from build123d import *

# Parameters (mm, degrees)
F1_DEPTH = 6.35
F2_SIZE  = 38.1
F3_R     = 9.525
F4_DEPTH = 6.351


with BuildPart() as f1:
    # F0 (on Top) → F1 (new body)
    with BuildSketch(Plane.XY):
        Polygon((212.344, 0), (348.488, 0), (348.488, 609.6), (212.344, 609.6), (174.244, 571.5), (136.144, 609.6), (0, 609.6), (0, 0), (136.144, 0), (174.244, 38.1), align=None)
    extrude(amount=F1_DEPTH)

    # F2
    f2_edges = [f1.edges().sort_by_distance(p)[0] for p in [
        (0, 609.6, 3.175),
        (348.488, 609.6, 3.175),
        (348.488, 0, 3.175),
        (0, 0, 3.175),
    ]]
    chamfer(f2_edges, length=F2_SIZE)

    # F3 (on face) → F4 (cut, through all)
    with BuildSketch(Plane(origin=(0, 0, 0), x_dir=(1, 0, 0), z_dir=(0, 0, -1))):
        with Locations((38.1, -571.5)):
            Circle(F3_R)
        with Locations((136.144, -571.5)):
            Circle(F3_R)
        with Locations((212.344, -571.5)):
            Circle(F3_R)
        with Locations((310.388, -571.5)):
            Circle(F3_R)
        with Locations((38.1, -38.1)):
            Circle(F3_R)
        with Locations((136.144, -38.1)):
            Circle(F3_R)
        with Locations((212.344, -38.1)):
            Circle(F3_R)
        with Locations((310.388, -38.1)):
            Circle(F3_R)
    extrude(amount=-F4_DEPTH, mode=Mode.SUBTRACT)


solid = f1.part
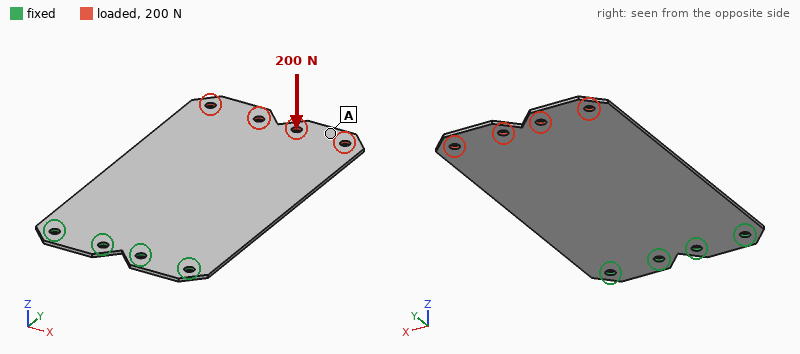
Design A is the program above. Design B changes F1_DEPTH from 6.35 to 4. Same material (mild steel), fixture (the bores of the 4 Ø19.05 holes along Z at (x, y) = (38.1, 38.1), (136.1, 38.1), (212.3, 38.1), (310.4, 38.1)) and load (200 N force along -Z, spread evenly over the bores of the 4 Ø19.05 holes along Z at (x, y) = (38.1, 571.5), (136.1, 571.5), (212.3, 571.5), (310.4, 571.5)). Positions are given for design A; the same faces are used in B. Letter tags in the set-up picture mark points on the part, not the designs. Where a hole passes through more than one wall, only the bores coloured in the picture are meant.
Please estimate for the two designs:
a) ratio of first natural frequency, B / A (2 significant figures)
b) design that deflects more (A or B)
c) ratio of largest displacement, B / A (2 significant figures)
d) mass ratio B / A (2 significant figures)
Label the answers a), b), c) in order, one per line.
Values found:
a) 0.63
b) B
c) 4.0
d) 0.63
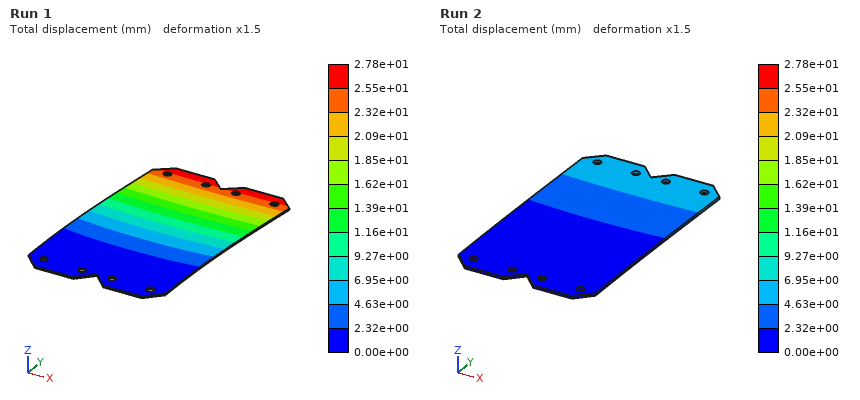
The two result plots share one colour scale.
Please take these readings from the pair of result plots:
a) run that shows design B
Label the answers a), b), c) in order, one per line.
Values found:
a) Run 1
